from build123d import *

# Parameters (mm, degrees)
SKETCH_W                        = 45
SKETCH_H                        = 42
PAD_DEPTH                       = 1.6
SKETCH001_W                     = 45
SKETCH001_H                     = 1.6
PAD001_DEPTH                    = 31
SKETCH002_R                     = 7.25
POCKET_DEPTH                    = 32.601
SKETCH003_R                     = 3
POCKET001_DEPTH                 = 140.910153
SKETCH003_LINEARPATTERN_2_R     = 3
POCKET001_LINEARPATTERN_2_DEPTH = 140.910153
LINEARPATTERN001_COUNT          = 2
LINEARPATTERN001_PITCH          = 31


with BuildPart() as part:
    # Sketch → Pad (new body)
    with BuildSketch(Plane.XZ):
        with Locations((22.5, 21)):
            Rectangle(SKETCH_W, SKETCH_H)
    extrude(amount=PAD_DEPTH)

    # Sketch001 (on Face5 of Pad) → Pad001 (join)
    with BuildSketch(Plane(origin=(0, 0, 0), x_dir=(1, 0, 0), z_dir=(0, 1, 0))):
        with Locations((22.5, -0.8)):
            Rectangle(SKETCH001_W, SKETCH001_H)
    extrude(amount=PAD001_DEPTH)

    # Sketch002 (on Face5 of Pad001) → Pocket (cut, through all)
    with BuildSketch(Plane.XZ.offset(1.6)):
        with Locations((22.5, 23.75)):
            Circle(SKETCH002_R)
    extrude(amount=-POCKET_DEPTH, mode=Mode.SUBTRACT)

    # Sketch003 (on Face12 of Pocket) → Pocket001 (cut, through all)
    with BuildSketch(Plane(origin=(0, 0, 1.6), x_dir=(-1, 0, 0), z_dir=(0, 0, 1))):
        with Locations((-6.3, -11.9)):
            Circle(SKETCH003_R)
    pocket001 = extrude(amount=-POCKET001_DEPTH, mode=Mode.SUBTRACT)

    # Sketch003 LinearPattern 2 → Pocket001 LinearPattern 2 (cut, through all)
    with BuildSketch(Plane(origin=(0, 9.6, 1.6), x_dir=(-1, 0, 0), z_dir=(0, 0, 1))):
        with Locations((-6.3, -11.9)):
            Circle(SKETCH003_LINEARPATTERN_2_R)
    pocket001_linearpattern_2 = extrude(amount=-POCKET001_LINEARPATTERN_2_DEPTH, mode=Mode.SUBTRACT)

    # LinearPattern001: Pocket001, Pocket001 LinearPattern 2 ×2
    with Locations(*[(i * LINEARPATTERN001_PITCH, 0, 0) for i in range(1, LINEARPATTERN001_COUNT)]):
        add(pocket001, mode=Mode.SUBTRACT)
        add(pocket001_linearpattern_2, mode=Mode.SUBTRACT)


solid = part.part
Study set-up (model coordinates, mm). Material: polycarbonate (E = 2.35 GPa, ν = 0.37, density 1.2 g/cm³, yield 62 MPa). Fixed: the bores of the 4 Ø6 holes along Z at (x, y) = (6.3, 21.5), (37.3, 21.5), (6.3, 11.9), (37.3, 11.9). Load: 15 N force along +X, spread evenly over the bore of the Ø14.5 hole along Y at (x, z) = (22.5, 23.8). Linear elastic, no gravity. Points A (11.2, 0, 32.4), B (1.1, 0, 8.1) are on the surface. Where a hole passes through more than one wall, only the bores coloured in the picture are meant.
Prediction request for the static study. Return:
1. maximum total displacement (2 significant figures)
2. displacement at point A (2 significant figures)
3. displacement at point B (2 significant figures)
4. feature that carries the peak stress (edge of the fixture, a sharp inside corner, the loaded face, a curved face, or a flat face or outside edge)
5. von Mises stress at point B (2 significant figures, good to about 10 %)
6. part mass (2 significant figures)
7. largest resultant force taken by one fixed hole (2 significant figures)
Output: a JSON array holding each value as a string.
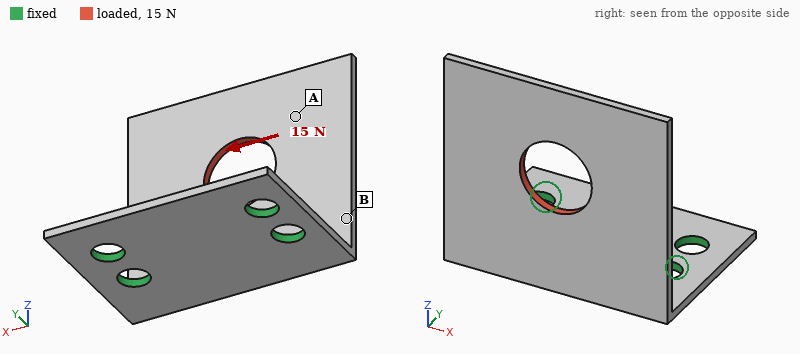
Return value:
["0.65 mm", "0.43 mm", "0.29 mm", "a flat face or outside edge", "3.2 MPa", "5.8 g", "14 N"]
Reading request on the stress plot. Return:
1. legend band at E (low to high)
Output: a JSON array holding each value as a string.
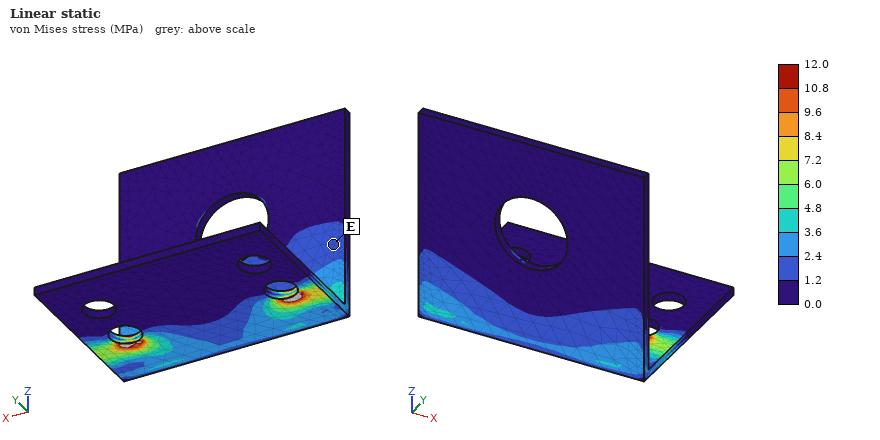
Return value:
["1.2 to 2.4 MPa"]
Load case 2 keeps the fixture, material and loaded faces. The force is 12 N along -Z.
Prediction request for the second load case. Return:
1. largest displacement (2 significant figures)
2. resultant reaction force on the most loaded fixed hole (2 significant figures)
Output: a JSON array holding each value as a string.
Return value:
["0.80 mm", "7.2 N"]
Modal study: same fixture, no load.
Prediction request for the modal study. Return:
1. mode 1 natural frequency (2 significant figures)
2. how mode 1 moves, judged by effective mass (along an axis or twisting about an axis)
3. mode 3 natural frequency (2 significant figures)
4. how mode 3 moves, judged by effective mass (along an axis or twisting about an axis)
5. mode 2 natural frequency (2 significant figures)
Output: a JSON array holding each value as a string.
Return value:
["160 Hz", "along Y", "620 Hz", "along X", "390 Hz"]
